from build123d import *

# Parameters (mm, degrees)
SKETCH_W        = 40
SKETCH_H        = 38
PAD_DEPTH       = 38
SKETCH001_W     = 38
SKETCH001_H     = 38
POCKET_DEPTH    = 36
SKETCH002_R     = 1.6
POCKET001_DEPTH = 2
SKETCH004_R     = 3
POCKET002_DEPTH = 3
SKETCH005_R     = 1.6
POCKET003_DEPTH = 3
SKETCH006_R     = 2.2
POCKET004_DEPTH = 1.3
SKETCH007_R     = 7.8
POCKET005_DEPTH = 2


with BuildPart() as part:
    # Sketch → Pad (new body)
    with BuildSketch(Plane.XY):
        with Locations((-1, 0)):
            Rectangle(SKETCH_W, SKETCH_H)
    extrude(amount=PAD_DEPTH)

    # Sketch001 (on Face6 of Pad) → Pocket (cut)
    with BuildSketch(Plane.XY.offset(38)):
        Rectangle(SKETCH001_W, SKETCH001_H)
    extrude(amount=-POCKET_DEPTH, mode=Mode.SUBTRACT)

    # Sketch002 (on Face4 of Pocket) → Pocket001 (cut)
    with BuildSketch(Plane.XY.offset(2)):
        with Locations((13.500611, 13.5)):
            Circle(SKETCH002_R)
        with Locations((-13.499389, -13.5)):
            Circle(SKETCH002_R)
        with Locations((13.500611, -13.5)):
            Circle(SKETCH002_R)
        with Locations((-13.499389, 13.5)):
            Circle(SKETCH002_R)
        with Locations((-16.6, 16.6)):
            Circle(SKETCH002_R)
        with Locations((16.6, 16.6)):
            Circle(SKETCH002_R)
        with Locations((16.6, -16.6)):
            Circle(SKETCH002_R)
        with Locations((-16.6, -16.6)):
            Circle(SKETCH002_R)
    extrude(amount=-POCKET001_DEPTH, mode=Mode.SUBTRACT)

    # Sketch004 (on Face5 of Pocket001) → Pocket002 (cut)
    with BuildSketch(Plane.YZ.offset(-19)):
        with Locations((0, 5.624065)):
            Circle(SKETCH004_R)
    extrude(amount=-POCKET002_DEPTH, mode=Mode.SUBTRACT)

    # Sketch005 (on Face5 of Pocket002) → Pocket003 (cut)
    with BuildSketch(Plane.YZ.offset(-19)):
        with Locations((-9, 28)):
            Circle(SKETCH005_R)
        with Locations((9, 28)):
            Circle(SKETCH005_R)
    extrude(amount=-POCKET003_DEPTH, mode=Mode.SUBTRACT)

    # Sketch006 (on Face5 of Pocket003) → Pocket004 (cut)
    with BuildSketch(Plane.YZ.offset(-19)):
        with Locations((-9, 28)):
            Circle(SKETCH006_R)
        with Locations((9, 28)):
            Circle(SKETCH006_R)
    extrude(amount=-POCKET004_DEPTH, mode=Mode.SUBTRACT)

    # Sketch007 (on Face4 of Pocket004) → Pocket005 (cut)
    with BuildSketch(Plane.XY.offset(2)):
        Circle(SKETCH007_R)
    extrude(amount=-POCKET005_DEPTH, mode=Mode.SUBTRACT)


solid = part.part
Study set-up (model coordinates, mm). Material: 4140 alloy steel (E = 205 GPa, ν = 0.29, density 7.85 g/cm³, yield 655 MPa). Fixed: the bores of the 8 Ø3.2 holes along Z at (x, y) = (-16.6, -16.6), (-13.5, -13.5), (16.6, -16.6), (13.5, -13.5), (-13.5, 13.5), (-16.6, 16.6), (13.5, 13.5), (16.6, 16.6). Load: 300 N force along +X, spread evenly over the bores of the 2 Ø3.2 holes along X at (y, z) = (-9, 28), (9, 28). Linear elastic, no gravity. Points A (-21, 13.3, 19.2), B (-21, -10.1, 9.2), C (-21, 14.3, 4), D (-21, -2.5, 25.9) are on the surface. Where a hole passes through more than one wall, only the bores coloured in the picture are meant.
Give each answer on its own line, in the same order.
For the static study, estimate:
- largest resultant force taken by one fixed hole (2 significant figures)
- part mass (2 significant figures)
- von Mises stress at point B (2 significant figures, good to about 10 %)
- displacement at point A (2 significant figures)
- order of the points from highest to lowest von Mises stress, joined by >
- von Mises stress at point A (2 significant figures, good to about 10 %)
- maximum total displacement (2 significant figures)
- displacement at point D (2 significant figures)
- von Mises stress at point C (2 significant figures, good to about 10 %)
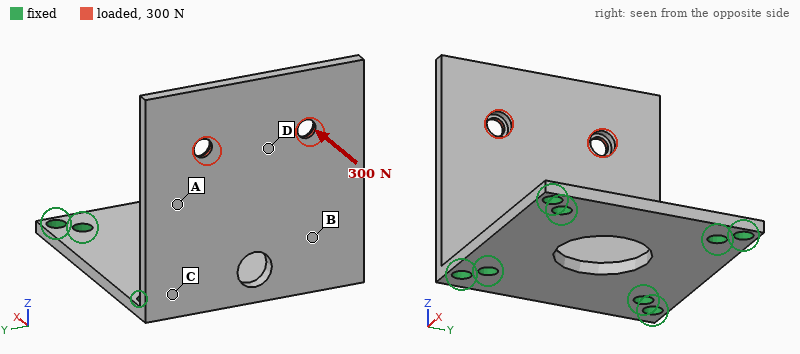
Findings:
490 N
40 g
220 MPa
0.29 mm
C > B > A > D
110 MPa
0.79 mm
0.47 mm
300 MPa
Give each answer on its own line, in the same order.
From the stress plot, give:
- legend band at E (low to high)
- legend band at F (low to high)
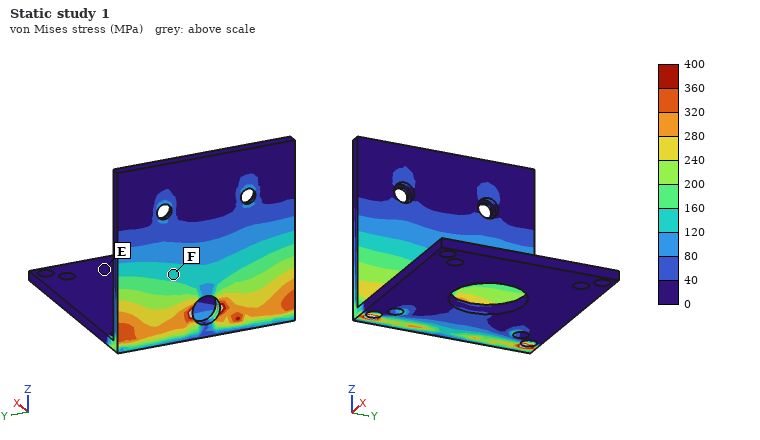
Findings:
0 to 40 MPa
120 to 160 MPa
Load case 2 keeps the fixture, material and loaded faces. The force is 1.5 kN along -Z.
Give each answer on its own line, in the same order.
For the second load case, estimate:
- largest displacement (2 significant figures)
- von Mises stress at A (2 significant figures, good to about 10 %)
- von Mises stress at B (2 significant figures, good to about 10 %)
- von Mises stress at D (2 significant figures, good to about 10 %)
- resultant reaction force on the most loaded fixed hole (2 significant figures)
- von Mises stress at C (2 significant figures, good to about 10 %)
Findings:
0.20 mm
61 MPa
60 MPa
38 MPa
830 N
76 MPa
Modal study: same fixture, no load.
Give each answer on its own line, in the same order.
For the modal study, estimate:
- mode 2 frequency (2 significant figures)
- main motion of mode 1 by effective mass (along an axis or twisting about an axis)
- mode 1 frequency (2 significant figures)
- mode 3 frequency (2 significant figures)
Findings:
2800 Hz
along X
1100 Hz
6600 Hz
